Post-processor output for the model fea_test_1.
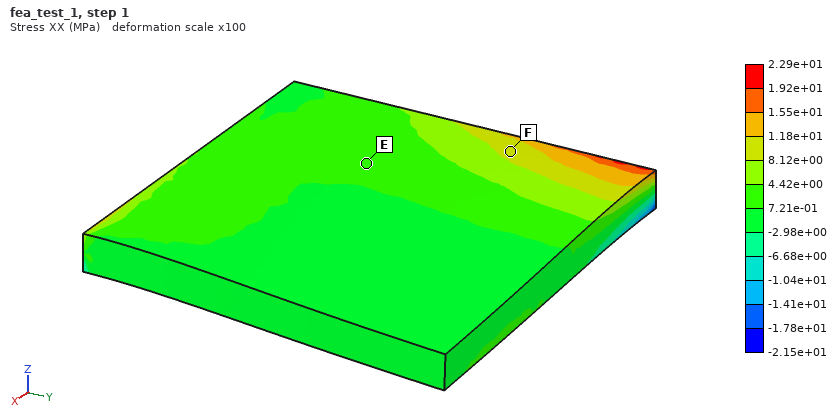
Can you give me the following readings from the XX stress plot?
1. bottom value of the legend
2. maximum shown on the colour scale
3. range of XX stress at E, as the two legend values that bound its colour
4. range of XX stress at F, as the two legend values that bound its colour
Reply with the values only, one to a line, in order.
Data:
-2.15e+01 MPa
2.29e+01 MPa
7.21e-01 to 4.42e+00 MPa
8.12e+00 to 1.18e+01 MPa
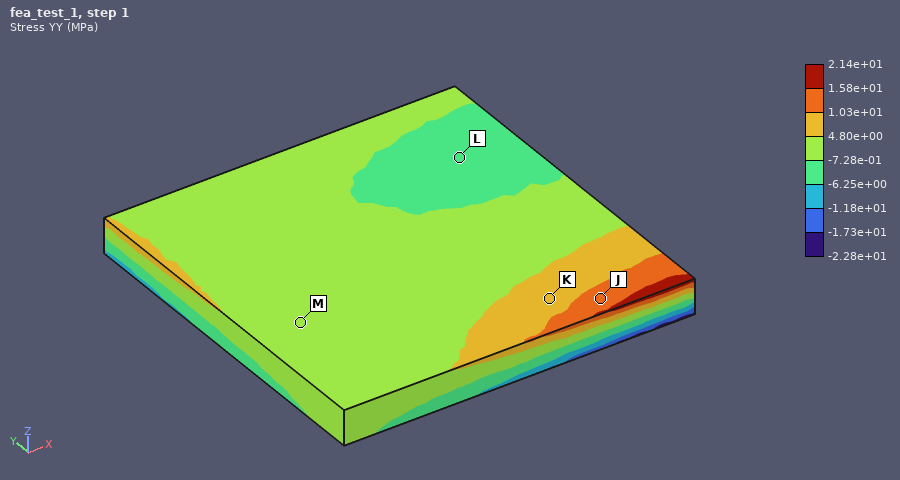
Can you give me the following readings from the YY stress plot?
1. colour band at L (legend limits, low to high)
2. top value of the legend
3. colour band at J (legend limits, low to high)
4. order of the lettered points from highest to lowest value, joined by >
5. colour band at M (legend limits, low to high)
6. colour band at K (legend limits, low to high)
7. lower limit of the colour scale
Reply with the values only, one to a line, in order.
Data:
-6.25e+00 to -7.28e-01 MPa
2.14e+01 MPa
1.03e+01 to 1.58e+01 MPa
J > K > M > L
-7.28e-01 to 4.80e+00 MPa
4.80e+00 to 1.03e+01 MPa
-2.28e+01 MPa
